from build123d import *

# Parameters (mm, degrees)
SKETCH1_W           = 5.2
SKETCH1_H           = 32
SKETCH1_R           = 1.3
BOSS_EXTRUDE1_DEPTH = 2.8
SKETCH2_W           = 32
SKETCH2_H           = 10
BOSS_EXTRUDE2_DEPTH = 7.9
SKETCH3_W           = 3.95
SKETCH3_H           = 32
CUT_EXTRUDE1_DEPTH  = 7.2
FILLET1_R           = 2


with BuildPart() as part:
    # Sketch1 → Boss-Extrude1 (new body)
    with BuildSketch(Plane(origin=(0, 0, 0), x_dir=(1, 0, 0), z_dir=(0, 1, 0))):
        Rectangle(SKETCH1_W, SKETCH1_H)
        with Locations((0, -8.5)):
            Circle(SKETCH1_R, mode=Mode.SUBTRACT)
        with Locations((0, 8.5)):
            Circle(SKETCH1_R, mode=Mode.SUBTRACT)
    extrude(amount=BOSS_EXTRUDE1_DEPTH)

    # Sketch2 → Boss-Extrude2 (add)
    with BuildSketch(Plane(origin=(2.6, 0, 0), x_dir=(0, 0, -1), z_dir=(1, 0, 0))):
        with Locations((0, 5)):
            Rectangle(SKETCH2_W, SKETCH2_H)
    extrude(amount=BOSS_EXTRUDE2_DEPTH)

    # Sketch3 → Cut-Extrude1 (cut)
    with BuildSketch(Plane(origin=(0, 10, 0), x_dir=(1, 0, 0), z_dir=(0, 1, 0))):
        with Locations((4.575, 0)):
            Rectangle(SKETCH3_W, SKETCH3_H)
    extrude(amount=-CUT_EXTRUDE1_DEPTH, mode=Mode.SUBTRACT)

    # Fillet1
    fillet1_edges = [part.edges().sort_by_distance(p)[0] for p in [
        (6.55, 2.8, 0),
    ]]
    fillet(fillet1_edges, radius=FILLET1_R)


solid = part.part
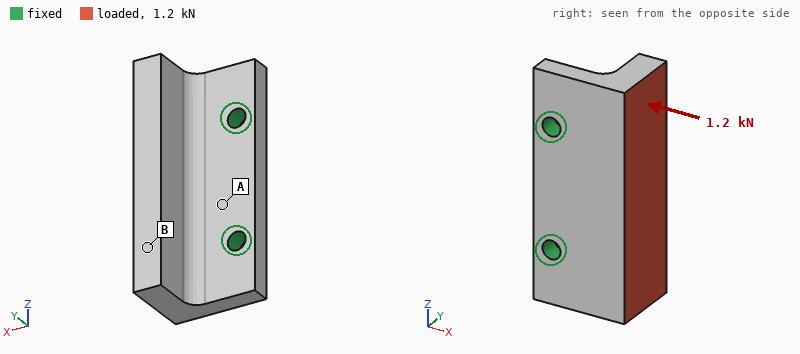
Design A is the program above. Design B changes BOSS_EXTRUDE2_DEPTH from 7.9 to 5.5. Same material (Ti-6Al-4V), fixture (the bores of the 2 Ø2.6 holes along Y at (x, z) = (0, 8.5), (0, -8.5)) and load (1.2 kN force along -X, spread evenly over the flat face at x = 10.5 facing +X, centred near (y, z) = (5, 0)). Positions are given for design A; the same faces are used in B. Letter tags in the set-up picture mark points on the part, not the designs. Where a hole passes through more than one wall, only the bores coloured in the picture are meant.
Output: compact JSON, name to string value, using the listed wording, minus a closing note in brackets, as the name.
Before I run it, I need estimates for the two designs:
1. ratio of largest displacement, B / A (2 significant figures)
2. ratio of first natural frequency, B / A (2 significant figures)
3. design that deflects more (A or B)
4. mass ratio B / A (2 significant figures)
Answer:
{"ratio of largest displacement, B / A": "1.3", "ratio of first natural frequency, B / A": "1.7", "design that deflects more": "B", "mass ratio B / A": "0.63"}
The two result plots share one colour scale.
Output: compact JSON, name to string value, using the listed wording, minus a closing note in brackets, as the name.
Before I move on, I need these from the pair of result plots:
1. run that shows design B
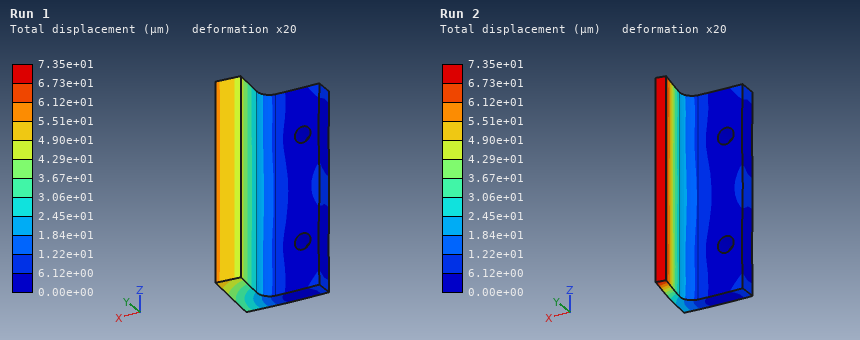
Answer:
{"run that shows design B": "Run 2"}
